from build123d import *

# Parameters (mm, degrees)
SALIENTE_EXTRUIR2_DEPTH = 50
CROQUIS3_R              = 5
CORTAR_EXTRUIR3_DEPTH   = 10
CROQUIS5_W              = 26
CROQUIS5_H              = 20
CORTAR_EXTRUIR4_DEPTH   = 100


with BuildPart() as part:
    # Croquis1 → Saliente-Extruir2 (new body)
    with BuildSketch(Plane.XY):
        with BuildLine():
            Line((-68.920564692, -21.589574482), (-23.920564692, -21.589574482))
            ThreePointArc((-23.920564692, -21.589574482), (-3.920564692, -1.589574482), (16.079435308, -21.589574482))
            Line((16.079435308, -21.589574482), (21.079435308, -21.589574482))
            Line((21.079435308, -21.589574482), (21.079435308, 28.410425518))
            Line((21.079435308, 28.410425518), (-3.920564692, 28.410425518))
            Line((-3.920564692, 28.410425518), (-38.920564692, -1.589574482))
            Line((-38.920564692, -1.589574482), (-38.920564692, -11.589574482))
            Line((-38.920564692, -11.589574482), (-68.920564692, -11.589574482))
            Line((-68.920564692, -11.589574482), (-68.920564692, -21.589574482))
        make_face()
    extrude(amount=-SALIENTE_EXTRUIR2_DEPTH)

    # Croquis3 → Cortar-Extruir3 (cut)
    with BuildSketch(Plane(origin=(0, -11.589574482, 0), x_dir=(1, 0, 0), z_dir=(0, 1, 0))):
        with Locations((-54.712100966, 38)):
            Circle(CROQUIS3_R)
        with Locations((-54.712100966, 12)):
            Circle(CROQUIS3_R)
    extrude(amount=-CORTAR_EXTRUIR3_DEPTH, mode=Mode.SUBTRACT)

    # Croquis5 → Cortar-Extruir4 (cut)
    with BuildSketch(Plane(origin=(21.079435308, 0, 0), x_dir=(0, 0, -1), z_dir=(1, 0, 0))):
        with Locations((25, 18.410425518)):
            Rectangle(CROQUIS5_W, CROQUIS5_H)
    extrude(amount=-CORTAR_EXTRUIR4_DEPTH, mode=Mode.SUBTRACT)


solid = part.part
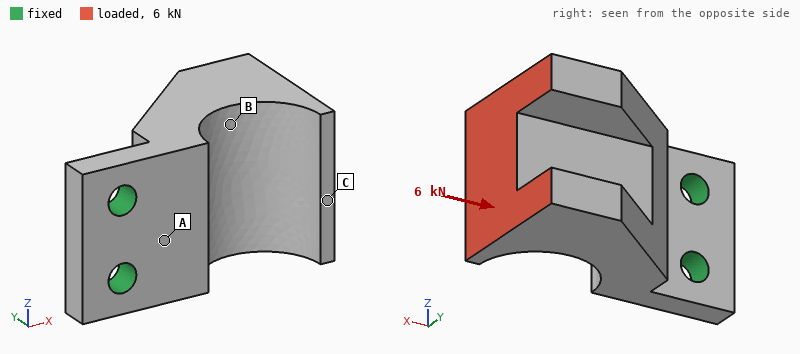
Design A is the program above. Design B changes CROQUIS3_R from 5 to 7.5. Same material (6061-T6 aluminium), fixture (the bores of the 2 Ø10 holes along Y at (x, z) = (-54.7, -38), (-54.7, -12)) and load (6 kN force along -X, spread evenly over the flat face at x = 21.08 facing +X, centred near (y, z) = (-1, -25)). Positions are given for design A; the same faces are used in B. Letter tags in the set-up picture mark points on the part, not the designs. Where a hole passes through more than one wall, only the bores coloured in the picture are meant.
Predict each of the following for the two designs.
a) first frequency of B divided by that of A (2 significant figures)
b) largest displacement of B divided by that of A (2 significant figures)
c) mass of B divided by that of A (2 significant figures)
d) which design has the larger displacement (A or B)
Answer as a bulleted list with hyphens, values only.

- 1.1
- 0.81
- 0.98
- A
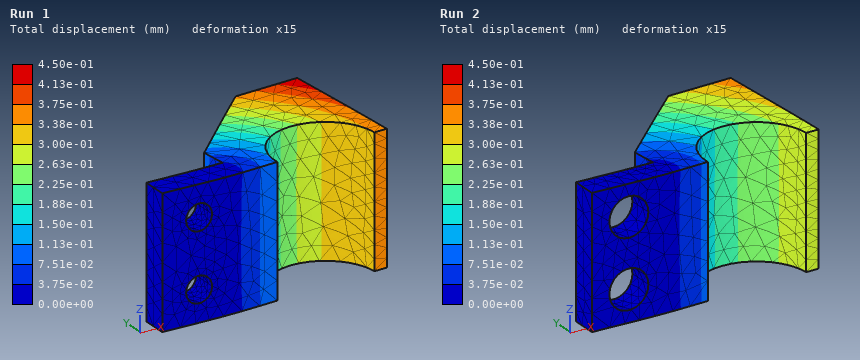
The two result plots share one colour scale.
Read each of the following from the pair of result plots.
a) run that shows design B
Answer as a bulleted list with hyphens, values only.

- Run 2
